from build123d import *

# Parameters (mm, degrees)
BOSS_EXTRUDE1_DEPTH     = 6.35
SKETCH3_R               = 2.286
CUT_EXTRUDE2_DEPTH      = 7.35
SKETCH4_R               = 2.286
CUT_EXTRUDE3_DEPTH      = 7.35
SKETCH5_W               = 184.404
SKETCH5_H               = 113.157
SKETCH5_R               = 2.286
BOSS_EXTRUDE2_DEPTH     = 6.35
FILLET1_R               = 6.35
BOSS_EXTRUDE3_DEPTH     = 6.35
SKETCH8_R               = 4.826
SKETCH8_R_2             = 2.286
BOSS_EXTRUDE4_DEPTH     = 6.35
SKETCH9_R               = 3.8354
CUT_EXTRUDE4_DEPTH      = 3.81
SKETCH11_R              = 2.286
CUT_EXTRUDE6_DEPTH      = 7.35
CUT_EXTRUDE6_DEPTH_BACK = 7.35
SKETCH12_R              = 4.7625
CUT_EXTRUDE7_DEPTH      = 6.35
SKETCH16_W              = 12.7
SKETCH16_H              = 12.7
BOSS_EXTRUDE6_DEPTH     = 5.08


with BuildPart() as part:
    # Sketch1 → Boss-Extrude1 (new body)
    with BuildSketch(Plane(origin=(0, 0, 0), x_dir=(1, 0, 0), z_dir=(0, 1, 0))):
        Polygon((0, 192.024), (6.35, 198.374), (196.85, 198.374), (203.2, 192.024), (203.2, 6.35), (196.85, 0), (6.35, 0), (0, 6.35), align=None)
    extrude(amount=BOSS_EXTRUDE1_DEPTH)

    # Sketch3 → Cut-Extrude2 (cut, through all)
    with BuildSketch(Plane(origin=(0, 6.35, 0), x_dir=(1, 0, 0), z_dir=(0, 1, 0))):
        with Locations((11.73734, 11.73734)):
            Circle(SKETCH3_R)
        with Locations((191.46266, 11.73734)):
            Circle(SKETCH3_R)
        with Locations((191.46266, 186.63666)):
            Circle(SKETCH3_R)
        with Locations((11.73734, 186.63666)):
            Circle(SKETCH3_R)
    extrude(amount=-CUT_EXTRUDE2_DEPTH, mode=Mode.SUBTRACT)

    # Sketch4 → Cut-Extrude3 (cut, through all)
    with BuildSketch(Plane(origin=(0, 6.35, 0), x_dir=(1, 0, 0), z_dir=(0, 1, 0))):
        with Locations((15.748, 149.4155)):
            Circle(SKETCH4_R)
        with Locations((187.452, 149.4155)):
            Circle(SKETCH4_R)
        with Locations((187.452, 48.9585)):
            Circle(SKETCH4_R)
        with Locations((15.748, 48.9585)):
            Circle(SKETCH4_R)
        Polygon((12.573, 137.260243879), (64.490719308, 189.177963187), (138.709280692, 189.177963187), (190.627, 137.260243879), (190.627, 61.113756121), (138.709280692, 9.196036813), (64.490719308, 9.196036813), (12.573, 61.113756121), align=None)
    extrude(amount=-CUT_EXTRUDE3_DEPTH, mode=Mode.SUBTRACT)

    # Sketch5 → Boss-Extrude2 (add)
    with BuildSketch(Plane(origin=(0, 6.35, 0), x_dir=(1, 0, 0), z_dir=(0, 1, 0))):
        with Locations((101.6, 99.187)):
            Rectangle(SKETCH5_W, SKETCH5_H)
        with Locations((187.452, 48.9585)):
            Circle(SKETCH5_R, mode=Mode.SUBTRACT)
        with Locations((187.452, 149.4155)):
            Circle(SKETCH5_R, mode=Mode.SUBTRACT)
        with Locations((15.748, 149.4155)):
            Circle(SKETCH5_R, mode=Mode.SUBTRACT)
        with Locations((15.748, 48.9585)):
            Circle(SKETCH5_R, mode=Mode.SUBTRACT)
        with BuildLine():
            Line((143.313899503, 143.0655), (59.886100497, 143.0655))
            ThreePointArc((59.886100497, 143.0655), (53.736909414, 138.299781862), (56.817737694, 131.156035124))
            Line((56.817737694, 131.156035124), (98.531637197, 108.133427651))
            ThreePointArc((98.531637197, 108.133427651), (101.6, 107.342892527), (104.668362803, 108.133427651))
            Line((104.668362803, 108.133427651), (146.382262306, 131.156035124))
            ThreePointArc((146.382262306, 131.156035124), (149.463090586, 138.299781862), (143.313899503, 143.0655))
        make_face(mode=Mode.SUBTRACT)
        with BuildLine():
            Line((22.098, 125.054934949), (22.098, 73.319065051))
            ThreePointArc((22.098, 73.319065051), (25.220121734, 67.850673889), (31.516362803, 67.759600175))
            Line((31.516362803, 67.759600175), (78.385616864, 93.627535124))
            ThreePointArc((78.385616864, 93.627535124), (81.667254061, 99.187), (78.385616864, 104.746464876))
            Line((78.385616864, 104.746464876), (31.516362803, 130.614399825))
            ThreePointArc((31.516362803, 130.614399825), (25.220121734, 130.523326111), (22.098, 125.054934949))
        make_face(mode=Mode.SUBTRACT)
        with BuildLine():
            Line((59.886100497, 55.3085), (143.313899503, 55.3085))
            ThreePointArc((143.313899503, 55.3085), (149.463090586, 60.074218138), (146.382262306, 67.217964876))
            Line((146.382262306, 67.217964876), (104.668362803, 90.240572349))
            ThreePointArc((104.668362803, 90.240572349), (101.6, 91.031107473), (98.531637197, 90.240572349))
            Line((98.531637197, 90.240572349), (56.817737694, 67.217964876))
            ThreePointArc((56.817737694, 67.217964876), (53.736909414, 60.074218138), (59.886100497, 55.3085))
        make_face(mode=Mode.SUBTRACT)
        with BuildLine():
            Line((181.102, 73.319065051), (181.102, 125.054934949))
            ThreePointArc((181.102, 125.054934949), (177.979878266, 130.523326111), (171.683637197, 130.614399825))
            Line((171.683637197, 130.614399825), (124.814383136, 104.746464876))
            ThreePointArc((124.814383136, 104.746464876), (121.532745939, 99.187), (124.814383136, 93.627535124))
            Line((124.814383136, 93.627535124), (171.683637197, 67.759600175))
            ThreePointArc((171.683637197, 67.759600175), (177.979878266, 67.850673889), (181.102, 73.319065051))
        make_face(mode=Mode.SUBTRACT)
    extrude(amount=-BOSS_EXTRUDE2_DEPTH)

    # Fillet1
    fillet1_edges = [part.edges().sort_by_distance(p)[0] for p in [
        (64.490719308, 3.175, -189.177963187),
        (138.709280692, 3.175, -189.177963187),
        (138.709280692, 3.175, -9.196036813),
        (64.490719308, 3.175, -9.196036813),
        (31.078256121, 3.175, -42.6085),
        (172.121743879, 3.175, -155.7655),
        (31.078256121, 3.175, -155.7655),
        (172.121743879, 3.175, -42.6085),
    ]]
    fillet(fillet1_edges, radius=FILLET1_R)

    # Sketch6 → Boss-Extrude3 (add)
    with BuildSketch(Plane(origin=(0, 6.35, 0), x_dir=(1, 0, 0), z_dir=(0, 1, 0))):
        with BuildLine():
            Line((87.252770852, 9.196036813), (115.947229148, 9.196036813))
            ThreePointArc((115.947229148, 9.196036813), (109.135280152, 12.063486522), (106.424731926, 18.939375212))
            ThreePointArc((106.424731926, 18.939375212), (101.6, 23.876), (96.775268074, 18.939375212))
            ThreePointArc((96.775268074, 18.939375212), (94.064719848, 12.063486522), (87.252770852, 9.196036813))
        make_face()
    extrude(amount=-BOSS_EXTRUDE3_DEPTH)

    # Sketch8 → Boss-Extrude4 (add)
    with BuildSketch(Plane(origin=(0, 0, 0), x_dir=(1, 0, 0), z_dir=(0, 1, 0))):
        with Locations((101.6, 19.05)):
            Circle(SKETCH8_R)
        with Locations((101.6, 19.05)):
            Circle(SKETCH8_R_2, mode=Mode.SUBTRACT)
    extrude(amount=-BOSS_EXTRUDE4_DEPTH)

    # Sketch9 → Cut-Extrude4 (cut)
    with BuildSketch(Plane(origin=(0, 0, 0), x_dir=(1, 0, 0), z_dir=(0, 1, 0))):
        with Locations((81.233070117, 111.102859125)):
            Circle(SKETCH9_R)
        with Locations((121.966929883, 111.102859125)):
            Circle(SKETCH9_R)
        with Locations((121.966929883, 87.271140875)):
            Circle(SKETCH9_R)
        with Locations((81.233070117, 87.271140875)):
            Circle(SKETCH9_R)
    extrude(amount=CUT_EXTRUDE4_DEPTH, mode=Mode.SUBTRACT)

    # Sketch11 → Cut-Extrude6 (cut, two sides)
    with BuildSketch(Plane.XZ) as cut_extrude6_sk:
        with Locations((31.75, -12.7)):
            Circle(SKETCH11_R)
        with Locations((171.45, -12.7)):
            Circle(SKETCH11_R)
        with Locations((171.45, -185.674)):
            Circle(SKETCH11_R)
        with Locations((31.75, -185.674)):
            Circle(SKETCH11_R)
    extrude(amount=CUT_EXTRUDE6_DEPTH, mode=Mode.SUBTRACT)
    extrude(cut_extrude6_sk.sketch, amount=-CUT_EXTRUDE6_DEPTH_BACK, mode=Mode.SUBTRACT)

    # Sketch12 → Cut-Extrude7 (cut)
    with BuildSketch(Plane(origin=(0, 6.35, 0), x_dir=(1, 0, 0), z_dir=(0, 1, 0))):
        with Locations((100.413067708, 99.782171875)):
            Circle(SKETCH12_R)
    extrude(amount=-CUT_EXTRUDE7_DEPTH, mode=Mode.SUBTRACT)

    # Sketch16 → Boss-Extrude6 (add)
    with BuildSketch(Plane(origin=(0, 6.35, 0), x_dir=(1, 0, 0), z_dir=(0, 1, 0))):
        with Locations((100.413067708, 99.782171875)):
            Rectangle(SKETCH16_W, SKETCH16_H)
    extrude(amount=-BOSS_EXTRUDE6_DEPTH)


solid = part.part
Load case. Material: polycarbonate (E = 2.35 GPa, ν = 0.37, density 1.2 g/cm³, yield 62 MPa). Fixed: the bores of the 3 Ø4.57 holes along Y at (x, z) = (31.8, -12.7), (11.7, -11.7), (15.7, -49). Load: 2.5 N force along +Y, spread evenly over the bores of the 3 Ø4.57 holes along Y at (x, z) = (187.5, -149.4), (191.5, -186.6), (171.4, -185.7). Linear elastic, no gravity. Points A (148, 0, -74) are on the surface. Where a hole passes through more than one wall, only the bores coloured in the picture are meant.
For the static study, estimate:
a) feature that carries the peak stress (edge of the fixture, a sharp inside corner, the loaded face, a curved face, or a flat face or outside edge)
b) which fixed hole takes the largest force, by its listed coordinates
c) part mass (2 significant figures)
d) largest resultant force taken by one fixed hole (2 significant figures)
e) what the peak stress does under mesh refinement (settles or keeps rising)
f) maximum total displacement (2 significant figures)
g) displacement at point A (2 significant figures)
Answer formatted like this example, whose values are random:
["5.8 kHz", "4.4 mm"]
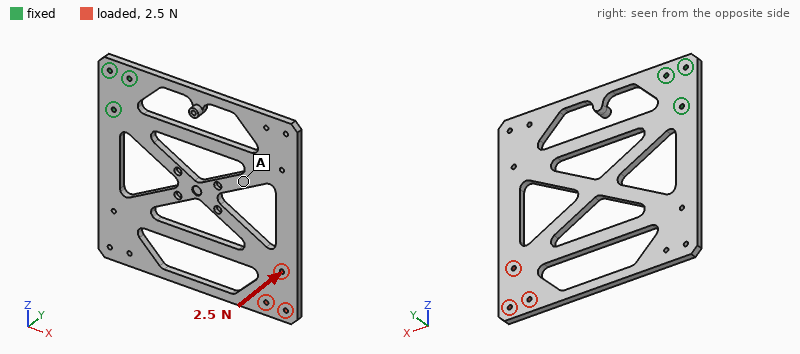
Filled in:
["edge of the fixture", "(15.7, -49)", "180 g", "6.1 N", "keeps rising", "3.3 mm", "1.1 mm"]
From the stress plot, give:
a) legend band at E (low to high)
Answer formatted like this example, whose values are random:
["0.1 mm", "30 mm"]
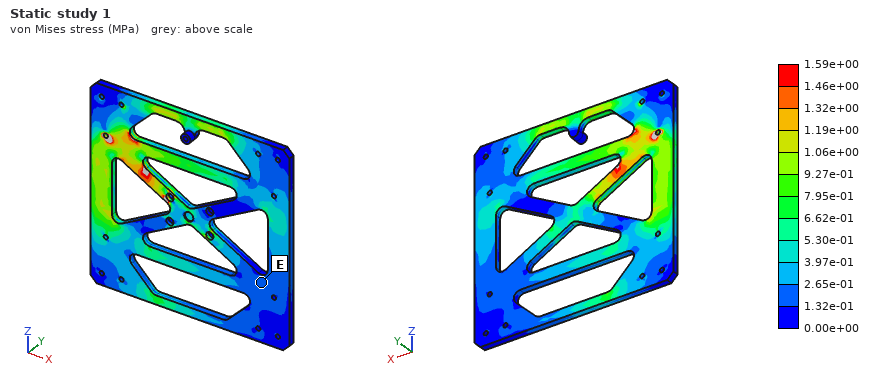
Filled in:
["1.32e-01 to 2.65e-01 MPa"]
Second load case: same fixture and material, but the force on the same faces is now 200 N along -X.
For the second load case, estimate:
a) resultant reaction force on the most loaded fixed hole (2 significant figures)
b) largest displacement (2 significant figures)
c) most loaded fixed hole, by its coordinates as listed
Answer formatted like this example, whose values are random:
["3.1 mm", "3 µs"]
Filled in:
["720 N", "3.3 mm", "(15.7, -49)"]
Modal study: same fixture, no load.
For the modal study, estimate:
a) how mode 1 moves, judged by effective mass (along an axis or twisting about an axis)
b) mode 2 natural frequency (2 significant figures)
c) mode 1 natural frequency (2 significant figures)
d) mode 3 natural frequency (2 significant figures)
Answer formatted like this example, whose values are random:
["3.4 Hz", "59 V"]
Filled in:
["along Y", "45 Hz", "23 Hz", "89 Hz"]
